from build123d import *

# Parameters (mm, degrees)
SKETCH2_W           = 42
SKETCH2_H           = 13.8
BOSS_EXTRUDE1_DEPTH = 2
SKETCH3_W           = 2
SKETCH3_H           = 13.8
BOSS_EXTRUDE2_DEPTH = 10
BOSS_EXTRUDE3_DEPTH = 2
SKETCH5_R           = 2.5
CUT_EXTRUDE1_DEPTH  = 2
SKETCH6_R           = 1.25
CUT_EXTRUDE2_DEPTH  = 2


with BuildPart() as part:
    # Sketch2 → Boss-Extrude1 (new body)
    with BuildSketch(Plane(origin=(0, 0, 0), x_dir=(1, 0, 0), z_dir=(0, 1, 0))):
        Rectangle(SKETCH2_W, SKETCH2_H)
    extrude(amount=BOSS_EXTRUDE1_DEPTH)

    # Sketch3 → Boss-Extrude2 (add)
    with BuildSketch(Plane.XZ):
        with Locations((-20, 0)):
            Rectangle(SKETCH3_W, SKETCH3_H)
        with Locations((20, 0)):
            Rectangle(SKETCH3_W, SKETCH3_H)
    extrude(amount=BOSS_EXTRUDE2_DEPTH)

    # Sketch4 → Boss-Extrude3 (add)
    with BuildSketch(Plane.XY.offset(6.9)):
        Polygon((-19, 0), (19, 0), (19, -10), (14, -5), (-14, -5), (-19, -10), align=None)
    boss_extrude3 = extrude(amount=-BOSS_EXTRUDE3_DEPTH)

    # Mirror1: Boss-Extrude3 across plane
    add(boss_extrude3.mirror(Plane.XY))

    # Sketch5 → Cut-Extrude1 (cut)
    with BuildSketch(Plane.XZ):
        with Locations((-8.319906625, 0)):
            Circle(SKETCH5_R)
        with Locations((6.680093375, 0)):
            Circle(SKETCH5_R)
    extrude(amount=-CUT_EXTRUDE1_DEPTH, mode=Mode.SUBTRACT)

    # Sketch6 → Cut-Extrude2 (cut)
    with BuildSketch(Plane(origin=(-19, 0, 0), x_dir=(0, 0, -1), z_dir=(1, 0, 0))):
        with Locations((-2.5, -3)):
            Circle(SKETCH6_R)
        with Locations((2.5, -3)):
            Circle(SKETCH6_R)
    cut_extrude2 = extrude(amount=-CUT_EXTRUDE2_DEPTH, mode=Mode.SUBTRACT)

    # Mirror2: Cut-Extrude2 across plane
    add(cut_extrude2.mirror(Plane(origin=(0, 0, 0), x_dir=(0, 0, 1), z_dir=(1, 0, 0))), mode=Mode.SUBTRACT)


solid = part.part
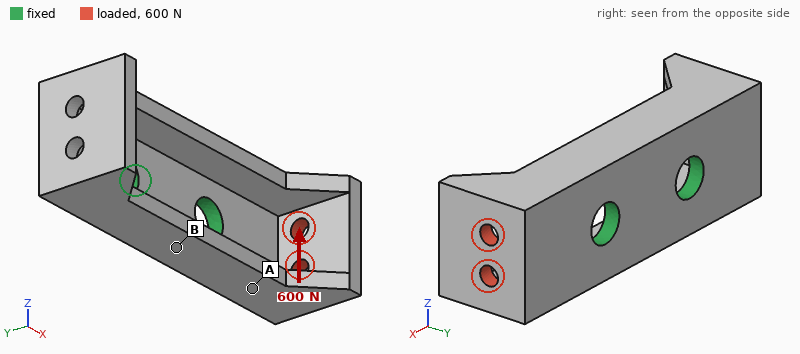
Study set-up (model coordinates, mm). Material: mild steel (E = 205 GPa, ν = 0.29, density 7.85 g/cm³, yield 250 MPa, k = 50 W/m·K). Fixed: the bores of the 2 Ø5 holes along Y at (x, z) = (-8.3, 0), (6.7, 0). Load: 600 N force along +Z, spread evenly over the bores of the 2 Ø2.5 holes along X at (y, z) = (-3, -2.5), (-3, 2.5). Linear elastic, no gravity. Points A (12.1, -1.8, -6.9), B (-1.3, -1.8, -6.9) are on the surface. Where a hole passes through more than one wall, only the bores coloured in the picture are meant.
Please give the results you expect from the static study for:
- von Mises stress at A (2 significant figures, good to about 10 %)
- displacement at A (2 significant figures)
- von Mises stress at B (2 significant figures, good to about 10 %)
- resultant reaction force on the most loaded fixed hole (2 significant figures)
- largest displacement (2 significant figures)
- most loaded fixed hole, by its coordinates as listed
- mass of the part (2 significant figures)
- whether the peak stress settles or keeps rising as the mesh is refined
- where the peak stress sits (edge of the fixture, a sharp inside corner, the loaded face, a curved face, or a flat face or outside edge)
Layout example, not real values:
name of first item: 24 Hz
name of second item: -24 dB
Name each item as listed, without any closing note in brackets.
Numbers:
von Mises stress at A: 76 MPa
displacement at A: 14 µm
von Mises stress at B: 22 MPa
resultant reaction force on the most loaded fixed hole: 820 N
largest displacement: 47 µm
most loaded fixed hole, by its coordinates as listed: (6.7, 0)
mass of the part: 19 g
whether the peak stress settles or keeps rising as the mesh is refined: keeps rising
where the peak stress sits: edge of the fixture
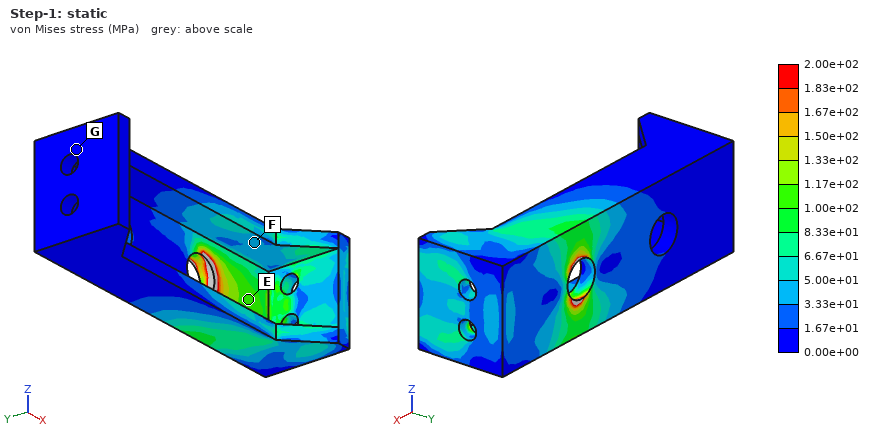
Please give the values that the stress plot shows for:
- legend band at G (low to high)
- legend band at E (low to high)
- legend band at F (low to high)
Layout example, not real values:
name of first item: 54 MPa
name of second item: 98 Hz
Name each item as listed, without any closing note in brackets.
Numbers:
legend band at G: 0.00e+00 to 1.67e+01 MPa
legend band at E: 1.00e+02 to 1.17e+02 MPa
legend band at F: 3.33e+01 to 5.00e+01 MPa
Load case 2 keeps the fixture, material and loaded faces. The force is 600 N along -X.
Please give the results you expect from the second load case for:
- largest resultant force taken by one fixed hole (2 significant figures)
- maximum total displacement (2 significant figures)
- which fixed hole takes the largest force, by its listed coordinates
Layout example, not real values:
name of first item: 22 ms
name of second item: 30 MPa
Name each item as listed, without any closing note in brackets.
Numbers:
largest resultant force taken by one fixed hole: 360 N
maximum total displacement: 13 µm
which fixed hole takes the largest force, by its listed coordinates: (6.7, 0)
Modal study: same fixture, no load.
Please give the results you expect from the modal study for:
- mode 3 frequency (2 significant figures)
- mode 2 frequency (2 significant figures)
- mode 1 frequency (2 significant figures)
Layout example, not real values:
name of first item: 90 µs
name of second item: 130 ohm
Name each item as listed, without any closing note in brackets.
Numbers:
mode 3 frequency: 10 kHz
mode 2 frequency: 10 kHz
mode 1 frequency: 9100 Hz
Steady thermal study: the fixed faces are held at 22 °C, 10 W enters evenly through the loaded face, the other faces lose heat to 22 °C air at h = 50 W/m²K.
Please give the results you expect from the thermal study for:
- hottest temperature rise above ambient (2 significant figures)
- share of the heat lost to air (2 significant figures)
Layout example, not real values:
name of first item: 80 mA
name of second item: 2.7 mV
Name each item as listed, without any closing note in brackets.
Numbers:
hottest temperature rise above ambient: 67 K
share of the heat lost to air: 20 %
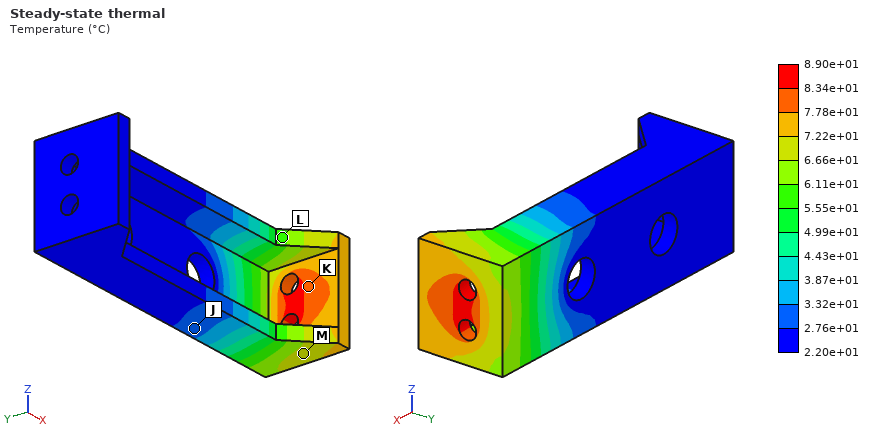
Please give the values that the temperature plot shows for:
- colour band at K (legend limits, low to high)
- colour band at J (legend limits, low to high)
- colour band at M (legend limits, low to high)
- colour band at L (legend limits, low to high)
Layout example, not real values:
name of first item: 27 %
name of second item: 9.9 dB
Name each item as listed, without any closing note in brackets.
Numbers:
colour band at K: 7.78e+01 to 8.34e+01 °C
colour band at J: 2.76e+01 to 3.32e+01 °C
colour band at M: 6.66e+01 to 7.22e+01 °C
colour band at L: 5.55e+01 to 6.11e+01 °C
